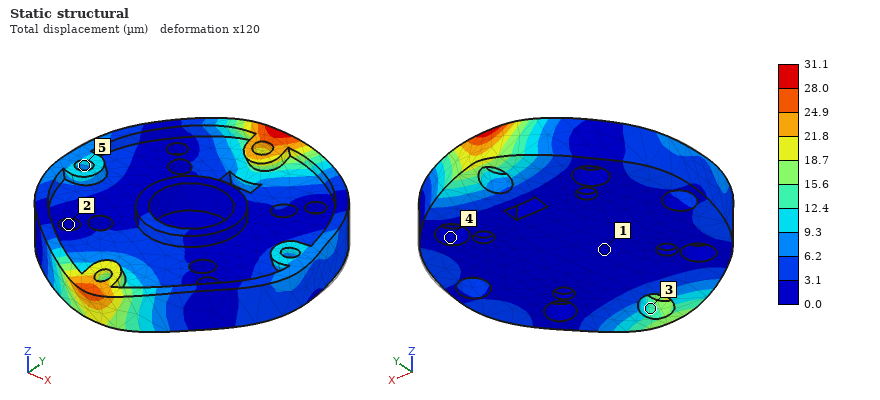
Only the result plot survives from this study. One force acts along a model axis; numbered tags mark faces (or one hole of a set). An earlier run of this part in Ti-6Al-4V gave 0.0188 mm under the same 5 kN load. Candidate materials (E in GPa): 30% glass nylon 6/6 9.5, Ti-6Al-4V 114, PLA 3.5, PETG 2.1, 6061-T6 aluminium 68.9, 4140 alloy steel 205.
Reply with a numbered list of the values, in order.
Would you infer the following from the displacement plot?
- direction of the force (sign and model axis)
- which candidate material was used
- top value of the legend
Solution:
1. -Y
2. 6061-T6 aluminium
3. 31.1 µm
